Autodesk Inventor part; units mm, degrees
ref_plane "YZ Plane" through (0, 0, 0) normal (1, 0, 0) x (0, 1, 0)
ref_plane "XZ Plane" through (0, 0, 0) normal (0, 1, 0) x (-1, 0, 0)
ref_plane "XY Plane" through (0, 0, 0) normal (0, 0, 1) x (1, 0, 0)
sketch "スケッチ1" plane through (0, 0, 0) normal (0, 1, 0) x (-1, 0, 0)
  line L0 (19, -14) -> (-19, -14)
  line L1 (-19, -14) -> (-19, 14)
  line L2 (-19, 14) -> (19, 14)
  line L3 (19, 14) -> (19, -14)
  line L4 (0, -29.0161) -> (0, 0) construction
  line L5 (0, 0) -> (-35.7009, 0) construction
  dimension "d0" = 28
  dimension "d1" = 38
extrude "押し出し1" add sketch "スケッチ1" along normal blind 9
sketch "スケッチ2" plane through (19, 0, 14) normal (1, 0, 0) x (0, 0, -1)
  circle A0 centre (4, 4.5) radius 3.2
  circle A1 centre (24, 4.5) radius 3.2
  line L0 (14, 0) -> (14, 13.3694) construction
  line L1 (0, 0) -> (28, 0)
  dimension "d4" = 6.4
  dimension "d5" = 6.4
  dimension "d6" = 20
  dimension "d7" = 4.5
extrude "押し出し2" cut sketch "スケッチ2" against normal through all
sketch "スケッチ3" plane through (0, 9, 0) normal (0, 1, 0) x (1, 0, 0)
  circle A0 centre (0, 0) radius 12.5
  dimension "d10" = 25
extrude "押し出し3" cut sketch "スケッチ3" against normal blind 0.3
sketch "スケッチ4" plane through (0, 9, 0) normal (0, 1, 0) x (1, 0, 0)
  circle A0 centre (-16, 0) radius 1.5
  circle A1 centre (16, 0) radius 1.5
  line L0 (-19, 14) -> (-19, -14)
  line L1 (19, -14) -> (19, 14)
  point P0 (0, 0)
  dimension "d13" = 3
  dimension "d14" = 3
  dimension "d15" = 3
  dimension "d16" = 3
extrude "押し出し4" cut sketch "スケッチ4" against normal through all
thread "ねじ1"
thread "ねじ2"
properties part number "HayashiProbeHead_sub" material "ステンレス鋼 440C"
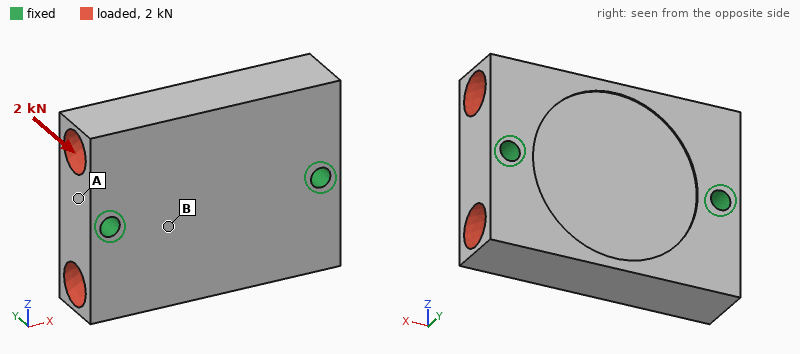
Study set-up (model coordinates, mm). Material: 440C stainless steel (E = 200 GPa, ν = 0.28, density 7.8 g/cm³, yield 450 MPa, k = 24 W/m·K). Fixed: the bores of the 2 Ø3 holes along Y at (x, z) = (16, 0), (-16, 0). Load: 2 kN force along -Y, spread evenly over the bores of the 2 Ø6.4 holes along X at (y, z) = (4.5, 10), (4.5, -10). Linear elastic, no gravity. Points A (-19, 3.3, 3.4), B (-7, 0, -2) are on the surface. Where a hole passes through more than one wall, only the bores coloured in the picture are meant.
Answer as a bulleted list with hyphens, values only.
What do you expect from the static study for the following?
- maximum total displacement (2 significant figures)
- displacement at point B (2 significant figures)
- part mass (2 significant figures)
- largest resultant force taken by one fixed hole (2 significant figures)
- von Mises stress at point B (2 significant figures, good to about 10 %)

- 5.4 µm
- 1.4 µm
- 53 g
- 1.0 kN
- 16 MPa
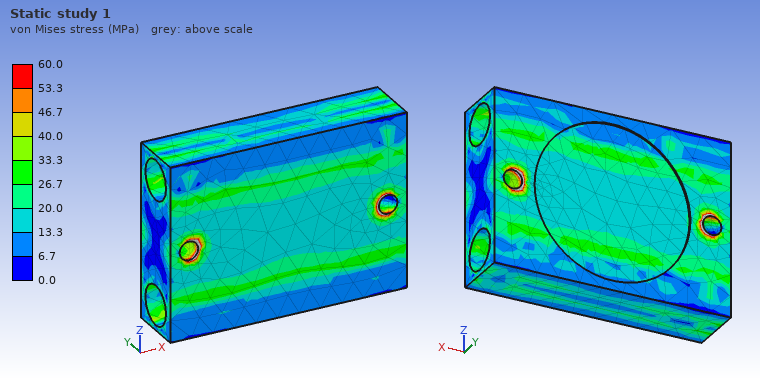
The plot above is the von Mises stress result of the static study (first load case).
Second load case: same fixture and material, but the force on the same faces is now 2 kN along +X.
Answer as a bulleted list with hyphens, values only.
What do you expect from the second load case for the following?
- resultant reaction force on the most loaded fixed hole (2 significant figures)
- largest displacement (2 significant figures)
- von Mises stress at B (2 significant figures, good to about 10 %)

- 1.0 kN
- 1.2 µm
- 5.5 MPa
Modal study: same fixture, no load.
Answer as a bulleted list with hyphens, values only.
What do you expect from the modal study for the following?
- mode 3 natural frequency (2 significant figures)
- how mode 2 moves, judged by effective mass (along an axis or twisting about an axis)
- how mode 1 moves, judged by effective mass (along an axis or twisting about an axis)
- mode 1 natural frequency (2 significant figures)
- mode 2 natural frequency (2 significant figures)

- 32 kHz
- along Y
- twisting about X
- 19 kHz
- 22 kHz
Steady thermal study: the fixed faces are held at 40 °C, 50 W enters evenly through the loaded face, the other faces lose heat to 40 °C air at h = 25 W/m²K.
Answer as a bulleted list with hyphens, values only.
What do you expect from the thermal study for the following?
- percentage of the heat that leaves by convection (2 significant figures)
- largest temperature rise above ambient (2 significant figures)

- 8.3 %
- 82 K
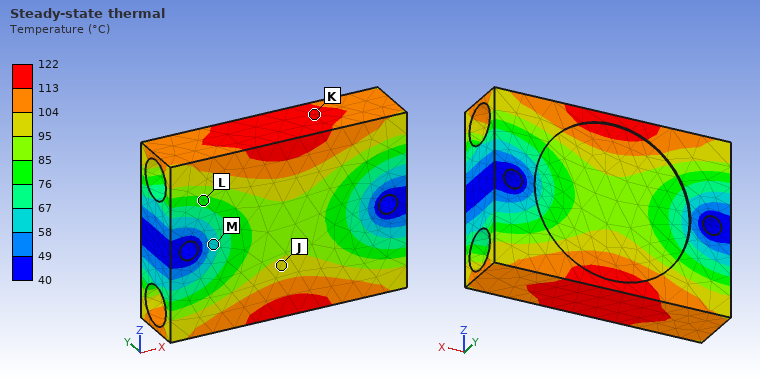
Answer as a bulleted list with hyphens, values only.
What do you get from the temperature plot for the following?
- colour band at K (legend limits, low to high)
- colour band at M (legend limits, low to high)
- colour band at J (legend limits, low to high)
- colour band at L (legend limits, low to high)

- 113 to 122 °C
- 58 to 67 °C
- 95 to 104 °C
- 76 to 85 °C
